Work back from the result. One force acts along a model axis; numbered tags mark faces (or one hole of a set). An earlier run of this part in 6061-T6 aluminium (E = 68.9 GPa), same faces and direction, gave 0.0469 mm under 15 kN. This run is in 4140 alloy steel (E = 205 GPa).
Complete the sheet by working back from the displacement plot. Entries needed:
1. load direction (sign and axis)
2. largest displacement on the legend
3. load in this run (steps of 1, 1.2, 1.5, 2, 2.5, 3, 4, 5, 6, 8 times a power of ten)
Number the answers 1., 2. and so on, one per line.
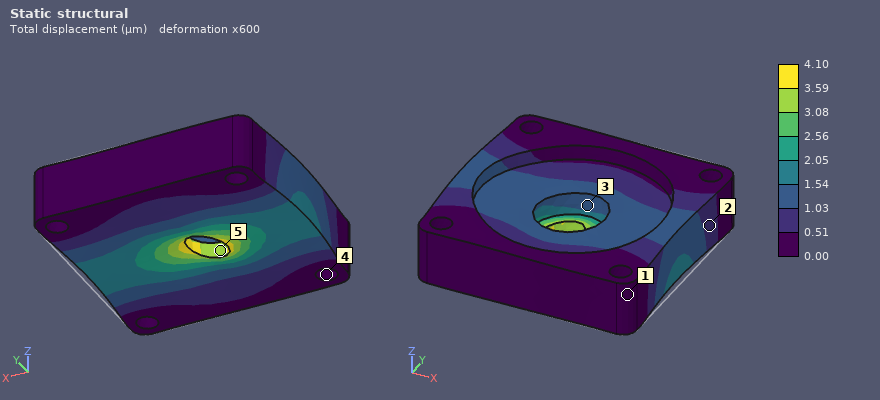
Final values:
1. -X
2. 4.10 µm
3. 4 kN
